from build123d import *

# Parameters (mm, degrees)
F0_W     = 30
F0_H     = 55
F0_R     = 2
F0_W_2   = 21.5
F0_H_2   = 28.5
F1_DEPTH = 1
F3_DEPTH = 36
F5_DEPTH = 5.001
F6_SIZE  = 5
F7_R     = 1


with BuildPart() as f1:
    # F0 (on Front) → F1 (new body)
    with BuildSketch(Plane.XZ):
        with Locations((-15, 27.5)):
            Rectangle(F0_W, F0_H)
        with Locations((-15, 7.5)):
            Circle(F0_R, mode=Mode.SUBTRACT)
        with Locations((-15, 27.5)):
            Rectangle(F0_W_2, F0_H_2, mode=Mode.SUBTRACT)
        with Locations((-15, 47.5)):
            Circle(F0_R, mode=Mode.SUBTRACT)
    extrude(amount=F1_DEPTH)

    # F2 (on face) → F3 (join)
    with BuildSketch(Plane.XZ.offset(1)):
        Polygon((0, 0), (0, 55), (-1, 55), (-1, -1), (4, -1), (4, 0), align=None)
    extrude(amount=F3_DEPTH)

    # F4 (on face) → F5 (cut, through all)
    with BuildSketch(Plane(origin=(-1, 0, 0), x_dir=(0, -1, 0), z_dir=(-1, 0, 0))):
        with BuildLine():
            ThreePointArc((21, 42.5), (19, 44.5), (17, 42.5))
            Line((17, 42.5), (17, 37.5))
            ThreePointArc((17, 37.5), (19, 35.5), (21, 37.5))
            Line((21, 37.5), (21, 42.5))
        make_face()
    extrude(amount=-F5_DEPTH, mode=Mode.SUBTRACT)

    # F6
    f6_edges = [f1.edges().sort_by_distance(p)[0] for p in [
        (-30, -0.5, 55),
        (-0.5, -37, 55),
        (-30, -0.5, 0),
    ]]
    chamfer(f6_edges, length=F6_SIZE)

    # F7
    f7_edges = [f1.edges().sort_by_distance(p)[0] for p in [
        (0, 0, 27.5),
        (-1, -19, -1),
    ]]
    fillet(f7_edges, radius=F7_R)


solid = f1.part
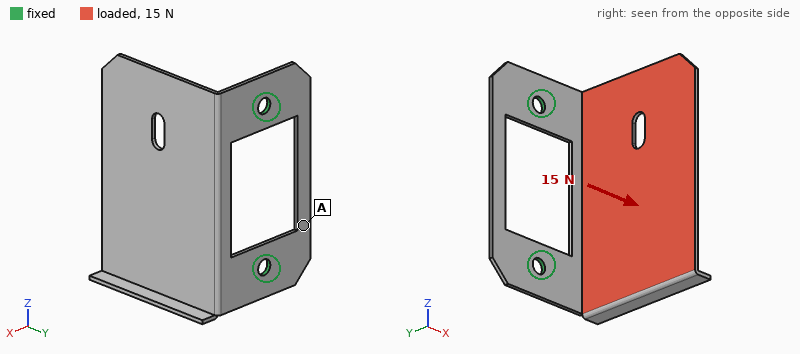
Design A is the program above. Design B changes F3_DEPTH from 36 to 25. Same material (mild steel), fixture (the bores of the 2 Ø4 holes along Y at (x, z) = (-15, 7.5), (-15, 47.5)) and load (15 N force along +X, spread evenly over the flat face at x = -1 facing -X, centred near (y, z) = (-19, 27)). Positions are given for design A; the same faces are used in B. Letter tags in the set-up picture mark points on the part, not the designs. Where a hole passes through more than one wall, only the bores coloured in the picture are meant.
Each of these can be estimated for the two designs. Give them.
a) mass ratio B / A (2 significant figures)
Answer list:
0.79
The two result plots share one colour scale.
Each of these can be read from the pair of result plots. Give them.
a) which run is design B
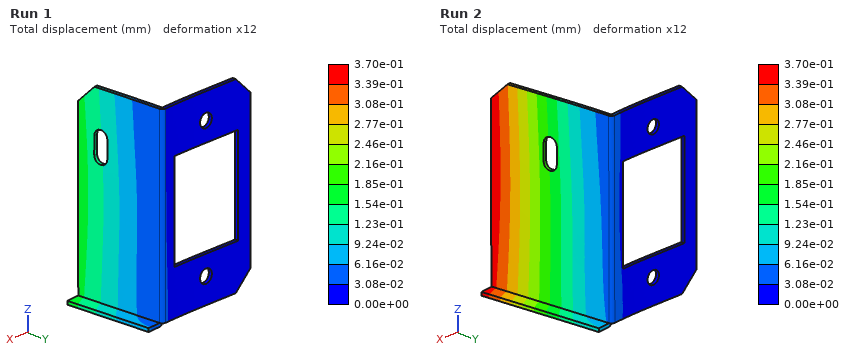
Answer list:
Run 1
